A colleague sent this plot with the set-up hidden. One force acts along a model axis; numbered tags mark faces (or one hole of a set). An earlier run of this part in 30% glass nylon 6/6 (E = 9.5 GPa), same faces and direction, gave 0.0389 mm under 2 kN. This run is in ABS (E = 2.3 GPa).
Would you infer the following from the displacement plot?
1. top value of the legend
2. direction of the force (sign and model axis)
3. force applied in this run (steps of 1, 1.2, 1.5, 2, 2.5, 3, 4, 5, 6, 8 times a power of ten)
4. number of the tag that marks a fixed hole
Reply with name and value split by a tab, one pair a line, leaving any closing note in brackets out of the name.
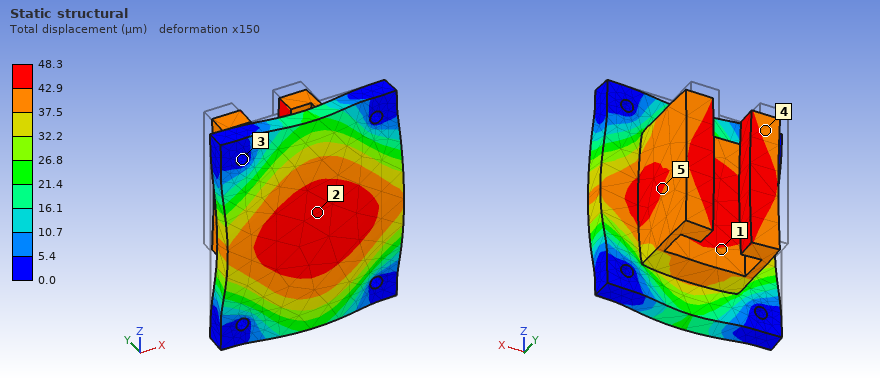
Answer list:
top value of the legend	48.3 µm
direction of the force	-Y
force applied in this run	600 N
number of the tag that marks a fixed hole	3
